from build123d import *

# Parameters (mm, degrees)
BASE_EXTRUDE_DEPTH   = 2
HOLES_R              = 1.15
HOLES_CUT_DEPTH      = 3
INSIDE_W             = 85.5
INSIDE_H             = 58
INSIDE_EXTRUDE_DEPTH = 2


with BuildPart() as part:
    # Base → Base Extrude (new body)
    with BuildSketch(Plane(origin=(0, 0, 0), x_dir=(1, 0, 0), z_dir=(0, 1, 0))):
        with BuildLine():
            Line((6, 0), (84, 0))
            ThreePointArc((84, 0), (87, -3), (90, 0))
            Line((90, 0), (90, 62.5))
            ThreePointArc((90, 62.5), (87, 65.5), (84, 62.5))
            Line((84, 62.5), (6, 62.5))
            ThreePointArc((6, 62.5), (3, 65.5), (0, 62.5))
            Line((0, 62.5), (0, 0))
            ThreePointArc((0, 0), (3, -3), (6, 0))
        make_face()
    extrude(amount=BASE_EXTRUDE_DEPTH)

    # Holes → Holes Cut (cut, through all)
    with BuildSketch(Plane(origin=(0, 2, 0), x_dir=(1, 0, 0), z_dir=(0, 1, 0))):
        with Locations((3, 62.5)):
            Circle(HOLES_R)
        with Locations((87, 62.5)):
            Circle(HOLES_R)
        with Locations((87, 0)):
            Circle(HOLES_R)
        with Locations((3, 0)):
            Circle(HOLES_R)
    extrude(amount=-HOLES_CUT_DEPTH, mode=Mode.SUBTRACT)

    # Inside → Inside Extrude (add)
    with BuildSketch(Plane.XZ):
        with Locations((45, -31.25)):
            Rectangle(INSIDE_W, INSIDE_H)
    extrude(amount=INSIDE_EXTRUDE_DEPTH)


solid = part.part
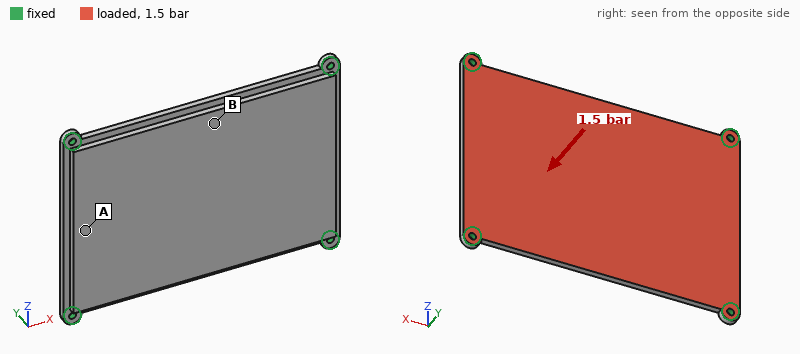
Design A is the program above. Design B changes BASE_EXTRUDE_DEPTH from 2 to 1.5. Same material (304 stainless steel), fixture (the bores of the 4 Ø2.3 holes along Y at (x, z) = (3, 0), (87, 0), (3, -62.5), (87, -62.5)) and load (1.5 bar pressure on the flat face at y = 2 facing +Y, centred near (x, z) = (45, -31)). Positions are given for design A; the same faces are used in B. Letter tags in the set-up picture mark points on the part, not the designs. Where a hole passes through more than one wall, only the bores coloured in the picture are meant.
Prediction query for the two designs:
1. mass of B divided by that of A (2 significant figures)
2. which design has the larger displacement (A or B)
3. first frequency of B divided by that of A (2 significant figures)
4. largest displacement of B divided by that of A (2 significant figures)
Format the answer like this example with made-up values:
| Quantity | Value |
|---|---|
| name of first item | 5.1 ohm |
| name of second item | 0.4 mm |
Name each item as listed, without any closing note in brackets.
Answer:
| Quantity | Value |
|---|---|
| mass of B divided by that of A | 0.87 |
| which design has the larger displacement | B |
| first frequency of B divided by that of A | 0.87 |
| largest displacement of B divided by that of A | 1.5 |
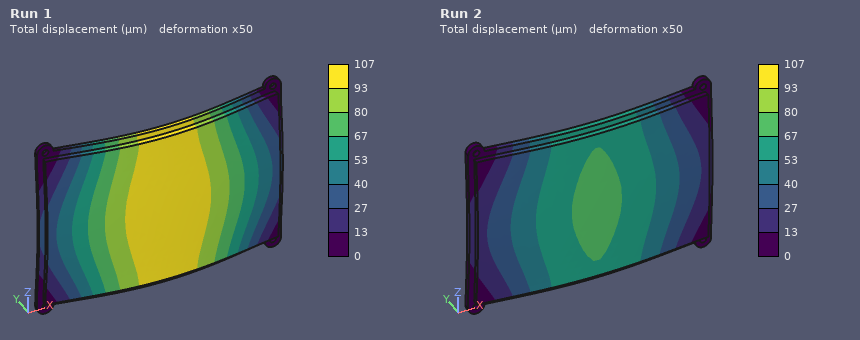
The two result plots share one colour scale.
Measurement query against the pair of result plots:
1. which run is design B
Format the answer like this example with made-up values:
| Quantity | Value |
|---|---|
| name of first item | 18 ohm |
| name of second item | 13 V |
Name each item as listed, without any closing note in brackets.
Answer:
| Quantity | Value |
|---|---|
| which run is design B | Run 1 |
